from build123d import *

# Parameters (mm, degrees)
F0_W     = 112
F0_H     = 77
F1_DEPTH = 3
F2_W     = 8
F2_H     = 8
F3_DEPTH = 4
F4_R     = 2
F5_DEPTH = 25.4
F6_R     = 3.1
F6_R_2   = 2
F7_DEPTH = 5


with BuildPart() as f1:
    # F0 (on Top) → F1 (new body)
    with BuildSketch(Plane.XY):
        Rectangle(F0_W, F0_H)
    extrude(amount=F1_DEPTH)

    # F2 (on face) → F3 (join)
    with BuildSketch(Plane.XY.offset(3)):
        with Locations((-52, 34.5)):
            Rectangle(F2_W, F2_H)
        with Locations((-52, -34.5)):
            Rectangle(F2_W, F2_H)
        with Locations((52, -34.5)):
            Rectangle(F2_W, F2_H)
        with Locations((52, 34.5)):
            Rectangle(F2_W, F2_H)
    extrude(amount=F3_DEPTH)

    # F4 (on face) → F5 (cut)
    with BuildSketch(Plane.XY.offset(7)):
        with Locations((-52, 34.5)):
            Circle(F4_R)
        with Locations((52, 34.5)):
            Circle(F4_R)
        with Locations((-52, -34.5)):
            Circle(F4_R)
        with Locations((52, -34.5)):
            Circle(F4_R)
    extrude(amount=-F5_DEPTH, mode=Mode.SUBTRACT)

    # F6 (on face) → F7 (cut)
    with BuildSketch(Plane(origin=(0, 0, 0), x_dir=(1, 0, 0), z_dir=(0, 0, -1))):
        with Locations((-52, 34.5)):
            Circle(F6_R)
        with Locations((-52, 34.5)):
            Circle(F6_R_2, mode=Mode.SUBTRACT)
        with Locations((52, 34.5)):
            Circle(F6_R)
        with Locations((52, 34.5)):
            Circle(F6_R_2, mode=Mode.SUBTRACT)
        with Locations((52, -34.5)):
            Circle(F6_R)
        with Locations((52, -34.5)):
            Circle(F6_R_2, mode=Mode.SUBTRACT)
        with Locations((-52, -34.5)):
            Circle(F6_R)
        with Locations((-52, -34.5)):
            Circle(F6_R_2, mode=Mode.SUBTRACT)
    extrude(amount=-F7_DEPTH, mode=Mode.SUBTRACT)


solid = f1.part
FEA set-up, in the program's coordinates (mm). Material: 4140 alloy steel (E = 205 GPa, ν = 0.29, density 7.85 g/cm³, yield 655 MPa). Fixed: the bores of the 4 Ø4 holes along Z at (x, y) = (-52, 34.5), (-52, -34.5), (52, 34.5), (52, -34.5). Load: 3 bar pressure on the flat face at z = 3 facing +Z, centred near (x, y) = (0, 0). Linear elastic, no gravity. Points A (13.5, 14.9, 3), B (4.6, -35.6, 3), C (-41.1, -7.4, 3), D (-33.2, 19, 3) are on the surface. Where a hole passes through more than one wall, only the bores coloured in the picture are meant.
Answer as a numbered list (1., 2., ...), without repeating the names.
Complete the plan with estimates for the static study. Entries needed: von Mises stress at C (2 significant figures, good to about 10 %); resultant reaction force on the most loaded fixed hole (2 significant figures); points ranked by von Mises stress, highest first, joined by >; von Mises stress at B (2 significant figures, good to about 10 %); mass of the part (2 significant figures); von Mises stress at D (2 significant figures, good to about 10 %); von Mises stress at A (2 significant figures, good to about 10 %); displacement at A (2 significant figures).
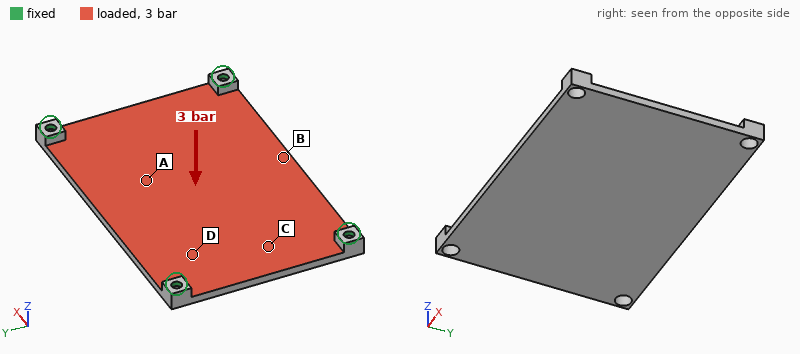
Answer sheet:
1. 53 MPa
2. 1.4 kN
3. B > A > C > D
4. 110 MPa
5. 210 g
6. 28 MPa
7. 79 MPa
8. 0.30 mm
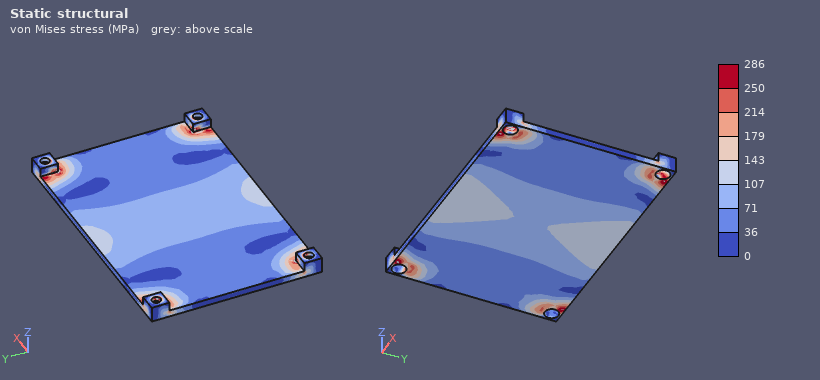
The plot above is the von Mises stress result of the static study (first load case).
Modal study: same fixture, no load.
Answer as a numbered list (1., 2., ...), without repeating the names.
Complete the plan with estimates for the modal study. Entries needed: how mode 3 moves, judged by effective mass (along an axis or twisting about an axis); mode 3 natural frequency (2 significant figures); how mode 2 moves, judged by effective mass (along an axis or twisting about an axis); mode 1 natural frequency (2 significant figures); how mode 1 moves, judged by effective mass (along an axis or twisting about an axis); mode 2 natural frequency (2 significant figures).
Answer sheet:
1. twisting about Y
2. 2700 Hz
3. twisting about X
4. 1100 Hz
5. along Z
6. 1900 Hz
